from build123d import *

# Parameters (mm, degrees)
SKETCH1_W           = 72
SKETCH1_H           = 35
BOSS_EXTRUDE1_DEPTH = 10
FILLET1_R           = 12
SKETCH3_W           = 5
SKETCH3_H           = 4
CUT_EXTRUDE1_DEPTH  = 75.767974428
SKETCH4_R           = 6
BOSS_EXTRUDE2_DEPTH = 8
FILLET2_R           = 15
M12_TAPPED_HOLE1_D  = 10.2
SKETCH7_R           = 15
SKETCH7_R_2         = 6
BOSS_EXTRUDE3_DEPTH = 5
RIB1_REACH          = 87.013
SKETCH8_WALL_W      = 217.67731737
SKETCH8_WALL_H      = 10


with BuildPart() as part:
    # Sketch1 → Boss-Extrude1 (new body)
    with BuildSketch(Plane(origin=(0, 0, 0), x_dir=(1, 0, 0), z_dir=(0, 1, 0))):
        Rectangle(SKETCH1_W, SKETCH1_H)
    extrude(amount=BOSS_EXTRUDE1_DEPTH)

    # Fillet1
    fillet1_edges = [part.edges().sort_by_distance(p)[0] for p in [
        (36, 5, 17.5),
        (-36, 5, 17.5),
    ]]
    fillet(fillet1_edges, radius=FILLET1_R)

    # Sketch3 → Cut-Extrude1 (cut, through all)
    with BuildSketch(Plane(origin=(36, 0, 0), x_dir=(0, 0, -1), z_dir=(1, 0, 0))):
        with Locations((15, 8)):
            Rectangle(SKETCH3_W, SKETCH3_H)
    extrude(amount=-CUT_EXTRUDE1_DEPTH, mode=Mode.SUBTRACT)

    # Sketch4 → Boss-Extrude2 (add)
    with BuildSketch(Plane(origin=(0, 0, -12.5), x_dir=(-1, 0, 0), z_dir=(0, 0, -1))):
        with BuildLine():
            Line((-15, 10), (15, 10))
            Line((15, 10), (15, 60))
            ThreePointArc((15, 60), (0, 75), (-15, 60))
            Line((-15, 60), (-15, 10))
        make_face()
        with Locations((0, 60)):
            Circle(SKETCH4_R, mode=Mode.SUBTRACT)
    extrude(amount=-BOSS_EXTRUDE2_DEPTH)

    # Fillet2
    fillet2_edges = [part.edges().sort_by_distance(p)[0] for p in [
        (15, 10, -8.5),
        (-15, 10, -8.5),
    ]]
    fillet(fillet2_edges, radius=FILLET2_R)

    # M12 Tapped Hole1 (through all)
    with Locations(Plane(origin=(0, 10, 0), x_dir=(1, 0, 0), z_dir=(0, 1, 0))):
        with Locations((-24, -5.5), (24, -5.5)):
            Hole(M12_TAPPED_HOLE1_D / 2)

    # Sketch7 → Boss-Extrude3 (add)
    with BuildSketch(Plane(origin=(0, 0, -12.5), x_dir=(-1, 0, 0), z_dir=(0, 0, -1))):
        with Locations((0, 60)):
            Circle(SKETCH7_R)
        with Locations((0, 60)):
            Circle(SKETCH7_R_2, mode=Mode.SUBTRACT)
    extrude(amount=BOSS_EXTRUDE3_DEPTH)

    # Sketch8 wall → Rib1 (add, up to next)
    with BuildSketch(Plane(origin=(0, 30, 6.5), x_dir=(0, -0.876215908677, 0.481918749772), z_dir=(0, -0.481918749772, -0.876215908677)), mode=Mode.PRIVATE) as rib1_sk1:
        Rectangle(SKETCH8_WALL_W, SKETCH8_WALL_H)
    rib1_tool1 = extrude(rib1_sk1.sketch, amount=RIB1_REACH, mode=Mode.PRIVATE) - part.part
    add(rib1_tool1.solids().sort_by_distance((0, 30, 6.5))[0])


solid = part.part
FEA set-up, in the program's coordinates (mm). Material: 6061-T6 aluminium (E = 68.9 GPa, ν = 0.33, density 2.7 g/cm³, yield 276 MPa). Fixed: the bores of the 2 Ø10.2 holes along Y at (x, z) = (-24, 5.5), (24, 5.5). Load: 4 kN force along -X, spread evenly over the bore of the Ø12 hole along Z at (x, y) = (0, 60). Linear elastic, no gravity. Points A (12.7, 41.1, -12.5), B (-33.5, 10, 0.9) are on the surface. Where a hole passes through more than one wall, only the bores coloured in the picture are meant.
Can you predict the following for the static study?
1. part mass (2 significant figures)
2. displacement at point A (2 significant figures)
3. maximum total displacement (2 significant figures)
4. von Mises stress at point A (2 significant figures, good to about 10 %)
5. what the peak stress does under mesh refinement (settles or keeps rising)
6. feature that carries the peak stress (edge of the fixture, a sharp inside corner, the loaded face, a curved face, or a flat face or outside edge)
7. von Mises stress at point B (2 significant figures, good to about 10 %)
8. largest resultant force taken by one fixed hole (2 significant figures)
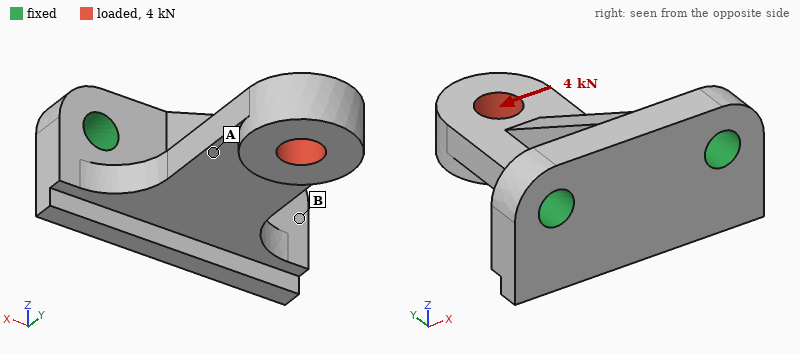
120 g
0.12 mm
0.28 mm
68 MPa
keeps rising
edge of the fixture
27 MPa
5.6 kN
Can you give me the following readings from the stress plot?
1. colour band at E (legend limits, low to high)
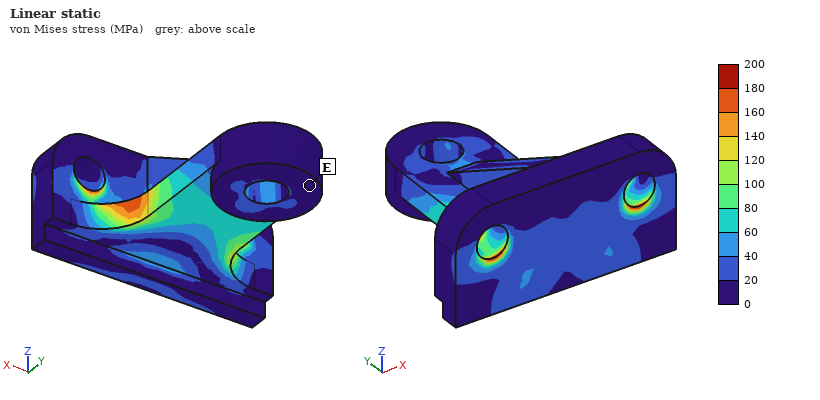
0 to 20 MPa
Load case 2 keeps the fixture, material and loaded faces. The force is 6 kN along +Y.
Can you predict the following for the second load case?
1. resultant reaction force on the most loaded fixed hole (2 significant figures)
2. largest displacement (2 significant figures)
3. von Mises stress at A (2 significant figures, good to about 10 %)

3.1 kN
0.25 mm
55 MPa
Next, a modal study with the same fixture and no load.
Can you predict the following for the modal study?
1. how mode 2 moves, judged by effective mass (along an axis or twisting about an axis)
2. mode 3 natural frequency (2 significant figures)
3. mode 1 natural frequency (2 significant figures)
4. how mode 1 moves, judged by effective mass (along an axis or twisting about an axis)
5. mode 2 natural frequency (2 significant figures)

along X
7600 Hz
2500 Hz
along Z
4300 Hz
